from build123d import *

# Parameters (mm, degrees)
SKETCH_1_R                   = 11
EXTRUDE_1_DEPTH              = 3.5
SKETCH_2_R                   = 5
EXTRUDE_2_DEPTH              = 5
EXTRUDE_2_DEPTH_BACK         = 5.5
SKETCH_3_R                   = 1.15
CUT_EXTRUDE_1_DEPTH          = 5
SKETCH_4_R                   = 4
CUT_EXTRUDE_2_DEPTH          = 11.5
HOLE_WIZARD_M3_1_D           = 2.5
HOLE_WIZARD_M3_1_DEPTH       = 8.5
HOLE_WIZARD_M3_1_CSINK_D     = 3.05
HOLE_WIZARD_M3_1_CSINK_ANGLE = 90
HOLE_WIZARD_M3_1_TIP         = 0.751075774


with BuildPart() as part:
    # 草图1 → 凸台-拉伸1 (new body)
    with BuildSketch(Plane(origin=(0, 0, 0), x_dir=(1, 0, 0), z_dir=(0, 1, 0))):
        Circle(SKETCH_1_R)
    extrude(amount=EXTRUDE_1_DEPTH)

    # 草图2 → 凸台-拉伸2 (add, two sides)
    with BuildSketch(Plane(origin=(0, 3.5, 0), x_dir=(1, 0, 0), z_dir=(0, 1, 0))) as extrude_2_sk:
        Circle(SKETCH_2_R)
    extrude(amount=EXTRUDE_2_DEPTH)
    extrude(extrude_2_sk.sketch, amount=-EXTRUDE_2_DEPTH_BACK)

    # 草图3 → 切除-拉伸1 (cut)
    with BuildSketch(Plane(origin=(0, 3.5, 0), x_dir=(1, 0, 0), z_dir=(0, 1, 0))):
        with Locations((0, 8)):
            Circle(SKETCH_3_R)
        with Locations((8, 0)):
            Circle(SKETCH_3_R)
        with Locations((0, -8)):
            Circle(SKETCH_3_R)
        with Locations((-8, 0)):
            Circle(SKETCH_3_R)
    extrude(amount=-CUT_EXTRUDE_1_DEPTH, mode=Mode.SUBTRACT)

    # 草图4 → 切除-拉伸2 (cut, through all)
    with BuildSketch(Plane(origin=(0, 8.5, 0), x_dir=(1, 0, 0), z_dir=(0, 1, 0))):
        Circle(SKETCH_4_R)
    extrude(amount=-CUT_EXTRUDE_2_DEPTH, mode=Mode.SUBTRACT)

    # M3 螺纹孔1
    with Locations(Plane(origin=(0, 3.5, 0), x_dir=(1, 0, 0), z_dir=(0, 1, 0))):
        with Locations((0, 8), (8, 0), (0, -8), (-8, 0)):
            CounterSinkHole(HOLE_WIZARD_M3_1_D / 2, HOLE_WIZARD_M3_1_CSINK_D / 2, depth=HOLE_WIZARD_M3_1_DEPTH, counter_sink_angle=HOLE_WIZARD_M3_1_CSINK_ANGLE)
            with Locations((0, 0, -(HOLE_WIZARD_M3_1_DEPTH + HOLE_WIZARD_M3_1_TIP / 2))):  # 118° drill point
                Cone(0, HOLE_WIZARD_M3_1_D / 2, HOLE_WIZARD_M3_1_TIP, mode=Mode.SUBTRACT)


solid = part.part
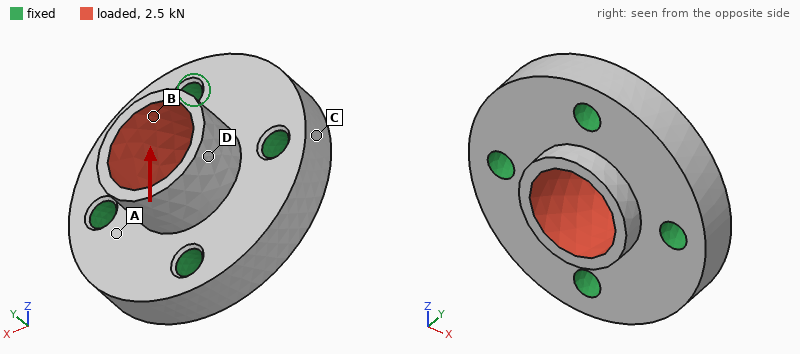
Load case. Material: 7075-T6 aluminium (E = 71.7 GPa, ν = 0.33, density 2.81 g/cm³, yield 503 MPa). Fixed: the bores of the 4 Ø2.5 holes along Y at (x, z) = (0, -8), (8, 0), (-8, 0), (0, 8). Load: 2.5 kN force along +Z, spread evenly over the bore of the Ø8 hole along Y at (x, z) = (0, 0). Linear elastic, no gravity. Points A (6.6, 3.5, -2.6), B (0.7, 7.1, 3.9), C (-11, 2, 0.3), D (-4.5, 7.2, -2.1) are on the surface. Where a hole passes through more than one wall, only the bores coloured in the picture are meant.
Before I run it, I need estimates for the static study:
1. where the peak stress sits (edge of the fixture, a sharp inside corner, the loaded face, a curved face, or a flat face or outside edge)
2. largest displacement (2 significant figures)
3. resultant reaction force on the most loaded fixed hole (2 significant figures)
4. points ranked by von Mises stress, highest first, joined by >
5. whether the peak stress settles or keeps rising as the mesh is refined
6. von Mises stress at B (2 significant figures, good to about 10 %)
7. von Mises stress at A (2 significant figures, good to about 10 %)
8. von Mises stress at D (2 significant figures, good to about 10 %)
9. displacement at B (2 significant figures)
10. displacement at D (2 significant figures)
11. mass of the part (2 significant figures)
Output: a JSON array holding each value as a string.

["edge of the fixture", "16 µm", "750 N", "B > D > A > C", "keeps rising", "54 MPa", "21 MPa", "35 MPa", "13 µm", "12 µm", "3.6 g"]
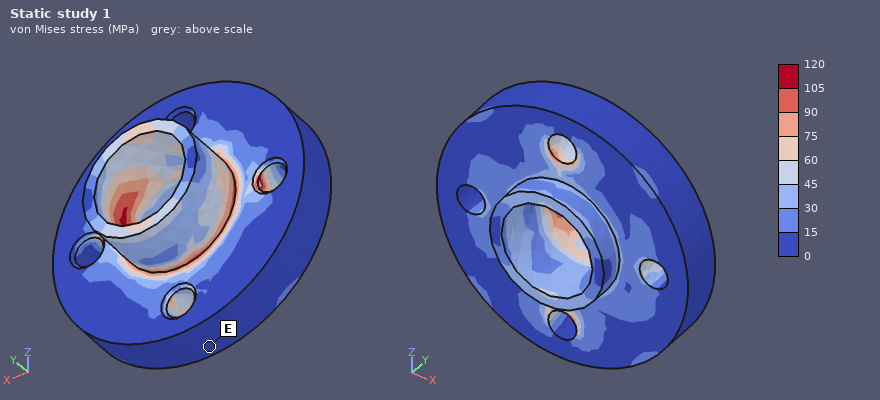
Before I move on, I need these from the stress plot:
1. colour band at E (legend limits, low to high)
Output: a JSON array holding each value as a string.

["0 to 15 MPa"]
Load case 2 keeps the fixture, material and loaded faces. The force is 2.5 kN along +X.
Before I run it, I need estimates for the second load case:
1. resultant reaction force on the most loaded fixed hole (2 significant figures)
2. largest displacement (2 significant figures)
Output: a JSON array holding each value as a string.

["750 N", "16 µm"]
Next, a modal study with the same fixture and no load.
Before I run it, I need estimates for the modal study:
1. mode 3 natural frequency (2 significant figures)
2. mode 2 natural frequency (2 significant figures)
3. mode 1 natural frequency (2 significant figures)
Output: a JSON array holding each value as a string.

["74 kHz", "71 kHz", "64 kHz"]
